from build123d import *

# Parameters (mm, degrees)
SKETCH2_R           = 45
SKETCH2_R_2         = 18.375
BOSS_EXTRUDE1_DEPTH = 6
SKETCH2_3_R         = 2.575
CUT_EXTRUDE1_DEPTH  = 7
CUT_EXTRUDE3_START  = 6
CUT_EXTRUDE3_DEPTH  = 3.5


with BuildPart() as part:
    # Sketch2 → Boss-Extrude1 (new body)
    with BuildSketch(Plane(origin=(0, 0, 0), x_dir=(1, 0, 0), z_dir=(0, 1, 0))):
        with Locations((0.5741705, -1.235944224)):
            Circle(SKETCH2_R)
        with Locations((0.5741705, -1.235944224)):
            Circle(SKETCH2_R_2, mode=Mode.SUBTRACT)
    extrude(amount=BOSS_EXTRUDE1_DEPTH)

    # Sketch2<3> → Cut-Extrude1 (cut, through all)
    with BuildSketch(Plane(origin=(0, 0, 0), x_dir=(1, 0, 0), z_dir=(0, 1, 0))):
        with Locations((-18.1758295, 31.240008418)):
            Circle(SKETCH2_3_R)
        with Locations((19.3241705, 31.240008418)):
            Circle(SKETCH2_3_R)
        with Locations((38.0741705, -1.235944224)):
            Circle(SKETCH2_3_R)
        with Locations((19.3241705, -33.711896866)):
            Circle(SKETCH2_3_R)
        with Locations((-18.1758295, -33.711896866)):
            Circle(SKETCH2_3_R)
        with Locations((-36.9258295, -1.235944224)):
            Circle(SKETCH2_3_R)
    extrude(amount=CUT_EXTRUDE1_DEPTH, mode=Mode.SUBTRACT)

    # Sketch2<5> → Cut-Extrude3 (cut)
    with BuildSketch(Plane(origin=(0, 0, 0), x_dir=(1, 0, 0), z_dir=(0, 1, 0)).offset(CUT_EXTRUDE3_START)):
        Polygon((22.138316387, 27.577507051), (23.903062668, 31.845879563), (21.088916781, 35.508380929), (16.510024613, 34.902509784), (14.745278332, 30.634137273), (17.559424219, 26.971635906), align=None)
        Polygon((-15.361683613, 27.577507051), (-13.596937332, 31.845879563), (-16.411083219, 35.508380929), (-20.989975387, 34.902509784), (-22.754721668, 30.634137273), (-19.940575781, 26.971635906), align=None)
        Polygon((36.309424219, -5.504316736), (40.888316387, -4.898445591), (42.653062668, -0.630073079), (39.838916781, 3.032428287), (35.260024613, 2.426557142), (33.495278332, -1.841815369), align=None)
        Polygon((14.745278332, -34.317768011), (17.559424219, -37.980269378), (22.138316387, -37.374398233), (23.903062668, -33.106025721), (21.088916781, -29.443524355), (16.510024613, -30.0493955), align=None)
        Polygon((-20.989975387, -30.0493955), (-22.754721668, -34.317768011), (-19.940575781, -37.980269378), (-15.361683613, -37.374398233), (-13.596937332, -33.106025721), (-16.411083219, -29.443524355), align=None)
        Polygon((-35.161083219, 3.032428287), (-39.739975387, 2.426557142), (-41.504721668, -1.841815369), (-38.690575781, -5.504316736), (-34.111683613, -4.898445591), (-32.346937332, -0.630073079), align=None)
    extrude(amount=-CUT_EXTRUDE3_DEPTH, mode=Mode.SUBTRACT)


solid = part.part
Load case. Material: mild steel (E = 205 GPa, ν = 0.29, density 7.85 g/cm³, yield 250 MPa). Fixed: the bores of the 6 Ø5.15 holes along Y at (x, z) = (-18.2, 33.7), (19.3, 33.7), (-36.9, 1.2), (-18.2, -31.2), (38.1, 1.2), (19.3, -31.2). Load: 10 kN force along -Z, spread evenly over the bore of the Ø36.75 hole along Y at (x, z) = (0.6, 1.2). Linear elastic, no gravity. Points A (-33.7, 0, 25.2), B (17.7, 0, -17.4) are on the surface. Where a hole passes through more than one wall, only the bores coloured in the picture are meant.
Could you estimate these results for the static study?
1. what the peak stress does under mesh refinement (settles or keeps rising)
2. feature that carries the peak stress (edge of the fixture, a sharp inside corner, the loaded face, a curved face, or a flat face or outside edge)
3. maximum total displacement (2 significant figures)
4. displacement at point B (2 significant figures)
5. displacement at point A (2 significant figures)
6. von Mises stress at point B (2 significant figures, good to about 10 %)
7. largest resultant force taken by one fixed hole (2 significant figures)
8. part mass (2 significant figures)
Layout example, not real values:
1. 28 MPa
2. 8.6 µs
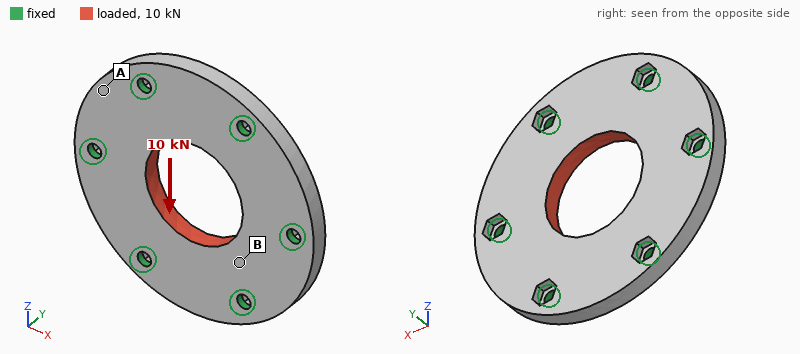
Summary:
1. keeps rising
2. edge of the fixture
3. 4.7 µm
4. 2.4 µm
5. 1.2 µm
6. 23 MPa
7. 1.9 kN
8. 240 g
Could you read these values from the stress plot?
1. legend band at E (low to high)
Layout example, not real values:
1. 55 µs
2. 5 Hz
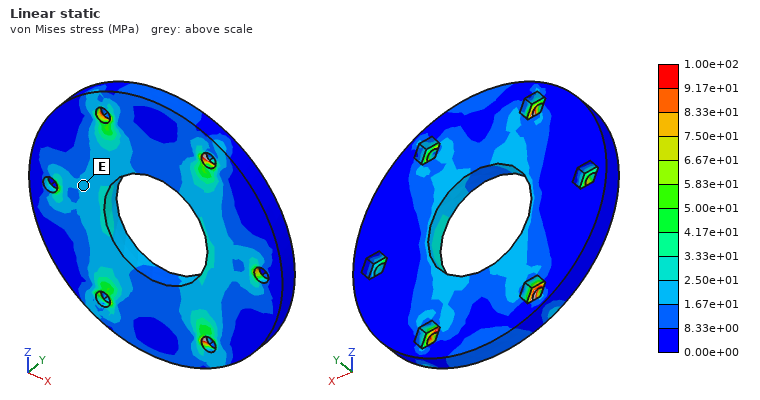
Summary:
1. 1.67e+01 to 2.50e+01 MPa
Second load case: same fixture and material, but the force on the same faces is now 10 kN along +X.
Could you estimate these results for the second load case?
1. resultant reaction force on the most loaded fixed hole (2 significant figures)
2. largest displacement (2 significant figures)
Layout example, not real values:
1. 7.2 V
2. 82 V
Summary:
1. 2.1 kN
2. 4.5 µm
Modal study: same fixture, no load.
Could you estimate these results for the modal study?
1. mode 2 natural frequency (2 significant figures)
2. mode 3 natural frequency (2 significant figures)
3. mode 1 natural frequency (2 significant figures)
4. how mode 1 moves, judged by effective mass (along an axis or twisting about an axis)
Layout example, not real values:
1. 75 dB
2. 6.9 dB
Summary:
1. 13 kHz
2. 13 kHz
3. 9300 Hz
4. along Y
